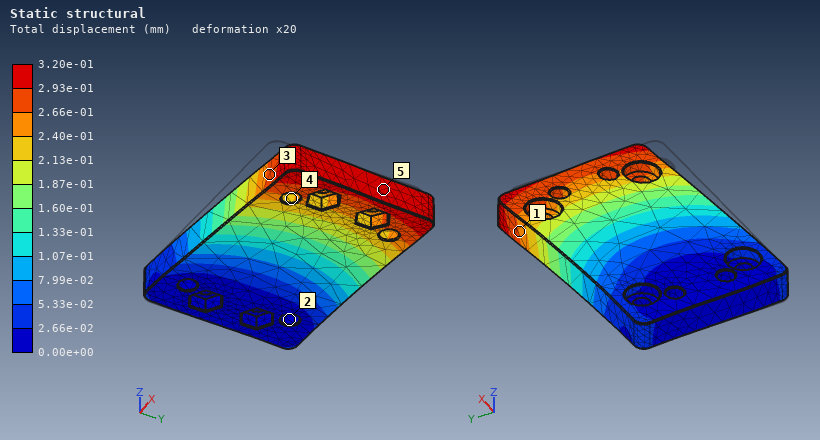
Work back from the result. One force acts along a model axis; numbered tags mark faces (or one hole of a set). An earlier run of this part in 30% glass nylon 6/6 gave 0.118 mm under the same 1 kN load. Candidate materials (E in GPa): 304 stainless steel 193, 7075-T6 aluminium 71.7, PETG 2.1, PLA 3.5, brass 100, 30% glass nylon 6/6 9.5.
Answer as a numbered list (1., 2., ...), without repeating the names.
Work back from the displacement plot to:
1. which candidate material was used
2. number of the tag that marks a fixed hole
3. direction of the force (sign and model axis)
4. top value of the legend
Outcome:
1. PLA
2. 2
3. +Y
4. 3.20e-01 mm
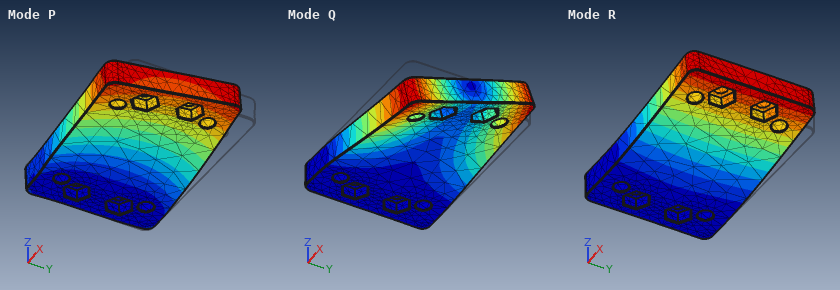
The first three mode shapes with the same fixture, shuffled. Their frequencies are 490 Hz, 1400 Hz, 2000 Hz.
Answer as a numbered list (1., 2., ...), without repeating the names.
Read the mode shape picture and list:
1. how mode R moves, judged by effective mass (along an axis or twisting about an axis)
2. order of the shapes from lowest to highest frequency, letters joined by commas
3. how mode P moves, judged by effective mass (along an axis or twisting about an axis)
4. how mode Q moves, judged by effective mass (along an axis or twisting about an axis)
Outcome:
1. along Z
2. R, Q, P
3. along Y
4. twisting about X
